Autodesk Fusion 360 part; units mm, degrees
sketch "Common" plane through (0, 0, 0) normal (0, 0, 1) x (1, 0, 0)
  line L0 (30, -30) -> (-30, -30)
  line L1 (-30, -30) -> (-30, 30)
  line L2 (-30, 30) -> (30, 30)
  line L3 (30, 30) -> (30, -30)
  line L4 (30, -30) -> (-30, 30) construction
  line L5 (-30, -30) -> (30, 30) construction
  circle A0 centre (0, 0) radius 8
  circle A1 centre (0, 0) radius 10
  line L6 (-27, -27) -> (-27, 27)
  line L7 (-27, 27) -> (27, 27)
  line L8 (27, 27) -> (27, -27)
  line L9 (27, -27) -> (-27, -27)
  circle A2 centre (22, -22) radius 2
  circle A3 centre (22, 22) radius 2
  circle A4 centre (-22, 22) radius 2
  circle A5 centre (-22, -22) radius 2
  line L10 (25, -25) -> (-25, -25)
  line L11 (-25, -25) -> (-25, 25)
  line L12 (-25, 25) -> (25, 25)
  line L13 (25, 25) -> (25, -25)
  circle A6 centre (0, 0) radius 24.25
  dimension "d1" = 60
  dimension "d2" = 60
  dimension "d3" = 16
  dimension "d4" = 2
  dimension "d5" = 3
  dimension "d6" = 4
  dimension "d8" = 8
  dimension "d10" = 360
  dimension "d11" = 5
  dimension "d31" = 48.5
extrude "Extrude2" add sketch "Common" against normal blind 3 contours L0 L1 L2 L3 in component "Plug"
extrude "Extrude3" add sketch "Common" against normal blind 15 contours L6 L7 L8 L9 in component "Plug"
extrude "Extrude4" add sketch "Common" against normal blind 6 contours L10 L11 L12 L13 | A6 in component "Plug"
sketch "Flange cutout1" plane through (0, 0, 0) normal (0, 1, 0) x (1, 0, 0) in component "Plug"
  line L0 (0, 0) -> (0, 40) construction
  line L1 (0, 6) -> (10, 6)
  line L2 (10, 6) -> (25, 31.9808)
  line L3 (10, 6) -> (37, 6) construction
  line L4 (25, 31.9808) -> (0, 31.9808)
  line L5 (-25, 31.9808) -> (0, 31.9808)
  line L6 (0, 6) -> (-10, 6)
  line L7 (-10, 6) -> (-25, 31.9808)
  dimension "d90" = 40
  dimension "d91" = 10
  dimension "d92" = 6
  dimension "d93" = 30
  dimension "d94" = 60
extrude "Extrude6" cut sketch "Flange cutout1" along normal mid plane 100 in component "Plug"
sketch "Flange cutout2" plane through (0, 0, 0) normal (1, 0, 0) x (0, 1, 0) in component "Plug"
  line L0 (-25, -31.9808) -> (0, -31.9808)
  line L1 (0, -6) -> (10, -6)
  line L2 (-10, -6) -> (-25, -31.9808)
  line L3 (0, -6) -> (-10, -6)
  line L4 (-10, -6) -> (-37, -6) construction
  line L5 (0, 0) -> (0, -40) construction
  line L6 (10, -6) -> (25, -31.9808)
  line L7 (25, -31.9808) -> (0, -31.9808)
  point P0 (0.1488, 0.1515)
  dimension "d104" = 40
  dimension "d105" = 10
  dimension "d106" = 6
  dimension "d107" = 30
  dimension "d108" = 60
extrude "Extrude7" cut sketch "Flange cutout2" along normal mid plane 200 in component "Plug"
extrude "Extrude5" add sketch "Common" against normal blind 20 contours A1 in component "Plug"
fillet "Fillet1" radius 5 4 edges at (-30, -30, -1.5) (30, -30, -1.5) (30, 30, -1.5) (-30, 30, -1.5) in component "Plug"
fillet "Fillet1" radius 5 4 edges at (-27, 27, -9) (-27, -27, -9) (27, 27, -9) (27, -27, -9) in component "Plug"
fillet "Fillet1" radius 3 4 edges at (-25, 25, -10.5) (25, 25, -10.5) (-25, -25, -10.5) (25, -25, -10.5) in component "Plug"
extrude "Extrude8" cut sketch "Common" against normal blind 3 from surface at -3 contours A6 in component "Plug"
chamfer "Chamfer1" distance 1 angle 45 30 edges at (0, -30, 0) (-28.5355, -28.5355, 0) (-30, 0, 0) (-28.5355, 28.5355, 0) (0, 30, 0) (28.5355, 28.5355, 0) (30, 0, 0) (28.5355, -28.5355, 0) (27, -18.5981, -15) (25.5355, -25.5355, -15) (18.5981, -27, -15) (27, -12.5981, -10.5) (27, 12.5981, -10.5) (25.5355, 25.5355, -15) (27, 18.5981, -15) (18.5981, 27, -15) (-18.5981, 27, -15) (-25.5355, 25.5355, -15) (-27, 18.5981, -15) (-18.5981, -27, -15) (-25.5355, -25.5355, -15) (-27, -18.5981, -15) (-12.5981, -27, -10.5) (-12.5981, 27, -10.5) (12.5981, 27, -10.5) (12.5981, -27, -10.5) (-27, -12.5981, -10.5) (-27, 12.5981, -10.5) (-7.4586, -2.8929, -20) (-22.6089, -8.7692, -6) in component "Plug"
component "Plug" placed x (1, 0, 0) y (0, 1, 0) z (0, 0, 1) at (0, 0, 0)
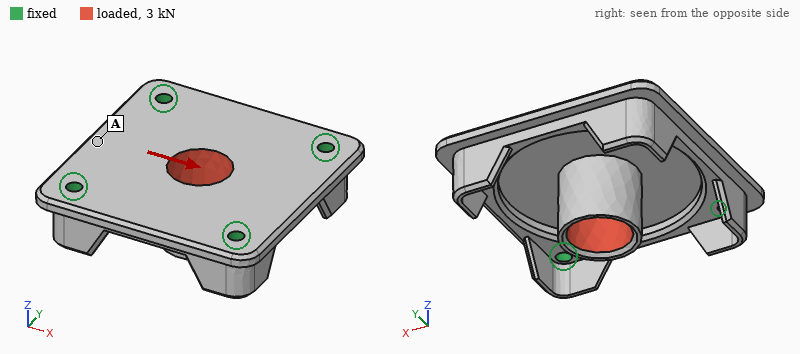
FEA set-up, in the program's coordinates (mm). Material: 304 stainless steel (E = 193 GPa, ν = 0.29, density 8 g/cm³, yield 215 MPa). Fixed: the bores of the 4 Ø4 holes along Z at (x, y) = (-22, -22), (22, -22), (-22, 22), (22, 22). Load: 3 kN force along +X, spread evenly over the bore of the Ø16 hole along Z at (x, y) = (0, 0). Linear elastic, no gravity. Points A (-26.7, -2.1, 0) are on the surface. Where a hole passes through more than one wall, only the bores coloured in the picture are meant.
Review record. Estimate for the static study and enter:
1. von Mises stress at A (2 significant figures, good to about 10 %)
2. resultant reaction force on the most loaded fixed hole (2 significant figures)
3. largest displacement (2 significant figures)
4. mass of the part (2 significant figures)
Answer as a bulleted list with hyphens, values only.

- 31 MPa
- 840 N
- 51 µm
- 130 g
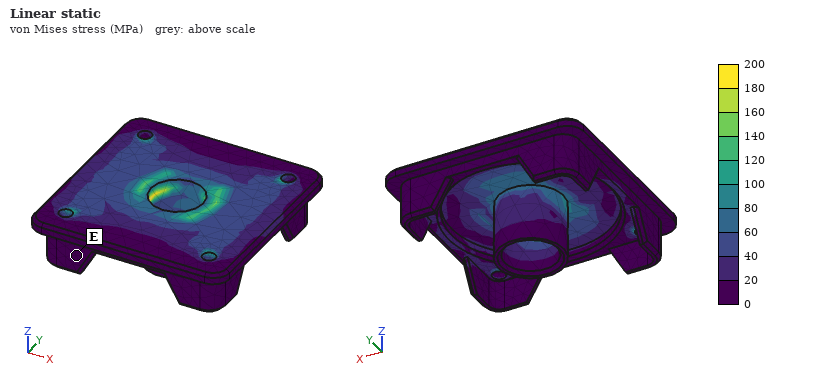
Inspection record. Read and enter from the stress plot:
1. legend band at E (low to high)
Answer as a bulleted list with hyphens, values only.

- 0 to 20 MPa
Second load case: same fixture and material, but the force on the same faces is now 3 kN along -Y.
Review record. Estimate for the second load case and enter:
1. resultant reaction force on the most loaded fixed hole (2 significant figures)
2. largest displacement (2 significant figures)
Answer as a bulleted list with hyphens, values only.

- 840 N
- 51 µm
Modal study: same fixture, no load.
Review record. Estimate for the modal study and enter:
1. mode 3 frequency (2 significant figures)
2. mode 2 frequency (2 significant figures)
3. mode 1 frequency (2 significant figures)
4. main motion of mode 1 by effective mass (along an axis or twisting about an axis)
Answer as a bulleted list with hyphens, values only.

- 8900 Hz
- 8900 Hz
- 7400 Hz
- along Z
